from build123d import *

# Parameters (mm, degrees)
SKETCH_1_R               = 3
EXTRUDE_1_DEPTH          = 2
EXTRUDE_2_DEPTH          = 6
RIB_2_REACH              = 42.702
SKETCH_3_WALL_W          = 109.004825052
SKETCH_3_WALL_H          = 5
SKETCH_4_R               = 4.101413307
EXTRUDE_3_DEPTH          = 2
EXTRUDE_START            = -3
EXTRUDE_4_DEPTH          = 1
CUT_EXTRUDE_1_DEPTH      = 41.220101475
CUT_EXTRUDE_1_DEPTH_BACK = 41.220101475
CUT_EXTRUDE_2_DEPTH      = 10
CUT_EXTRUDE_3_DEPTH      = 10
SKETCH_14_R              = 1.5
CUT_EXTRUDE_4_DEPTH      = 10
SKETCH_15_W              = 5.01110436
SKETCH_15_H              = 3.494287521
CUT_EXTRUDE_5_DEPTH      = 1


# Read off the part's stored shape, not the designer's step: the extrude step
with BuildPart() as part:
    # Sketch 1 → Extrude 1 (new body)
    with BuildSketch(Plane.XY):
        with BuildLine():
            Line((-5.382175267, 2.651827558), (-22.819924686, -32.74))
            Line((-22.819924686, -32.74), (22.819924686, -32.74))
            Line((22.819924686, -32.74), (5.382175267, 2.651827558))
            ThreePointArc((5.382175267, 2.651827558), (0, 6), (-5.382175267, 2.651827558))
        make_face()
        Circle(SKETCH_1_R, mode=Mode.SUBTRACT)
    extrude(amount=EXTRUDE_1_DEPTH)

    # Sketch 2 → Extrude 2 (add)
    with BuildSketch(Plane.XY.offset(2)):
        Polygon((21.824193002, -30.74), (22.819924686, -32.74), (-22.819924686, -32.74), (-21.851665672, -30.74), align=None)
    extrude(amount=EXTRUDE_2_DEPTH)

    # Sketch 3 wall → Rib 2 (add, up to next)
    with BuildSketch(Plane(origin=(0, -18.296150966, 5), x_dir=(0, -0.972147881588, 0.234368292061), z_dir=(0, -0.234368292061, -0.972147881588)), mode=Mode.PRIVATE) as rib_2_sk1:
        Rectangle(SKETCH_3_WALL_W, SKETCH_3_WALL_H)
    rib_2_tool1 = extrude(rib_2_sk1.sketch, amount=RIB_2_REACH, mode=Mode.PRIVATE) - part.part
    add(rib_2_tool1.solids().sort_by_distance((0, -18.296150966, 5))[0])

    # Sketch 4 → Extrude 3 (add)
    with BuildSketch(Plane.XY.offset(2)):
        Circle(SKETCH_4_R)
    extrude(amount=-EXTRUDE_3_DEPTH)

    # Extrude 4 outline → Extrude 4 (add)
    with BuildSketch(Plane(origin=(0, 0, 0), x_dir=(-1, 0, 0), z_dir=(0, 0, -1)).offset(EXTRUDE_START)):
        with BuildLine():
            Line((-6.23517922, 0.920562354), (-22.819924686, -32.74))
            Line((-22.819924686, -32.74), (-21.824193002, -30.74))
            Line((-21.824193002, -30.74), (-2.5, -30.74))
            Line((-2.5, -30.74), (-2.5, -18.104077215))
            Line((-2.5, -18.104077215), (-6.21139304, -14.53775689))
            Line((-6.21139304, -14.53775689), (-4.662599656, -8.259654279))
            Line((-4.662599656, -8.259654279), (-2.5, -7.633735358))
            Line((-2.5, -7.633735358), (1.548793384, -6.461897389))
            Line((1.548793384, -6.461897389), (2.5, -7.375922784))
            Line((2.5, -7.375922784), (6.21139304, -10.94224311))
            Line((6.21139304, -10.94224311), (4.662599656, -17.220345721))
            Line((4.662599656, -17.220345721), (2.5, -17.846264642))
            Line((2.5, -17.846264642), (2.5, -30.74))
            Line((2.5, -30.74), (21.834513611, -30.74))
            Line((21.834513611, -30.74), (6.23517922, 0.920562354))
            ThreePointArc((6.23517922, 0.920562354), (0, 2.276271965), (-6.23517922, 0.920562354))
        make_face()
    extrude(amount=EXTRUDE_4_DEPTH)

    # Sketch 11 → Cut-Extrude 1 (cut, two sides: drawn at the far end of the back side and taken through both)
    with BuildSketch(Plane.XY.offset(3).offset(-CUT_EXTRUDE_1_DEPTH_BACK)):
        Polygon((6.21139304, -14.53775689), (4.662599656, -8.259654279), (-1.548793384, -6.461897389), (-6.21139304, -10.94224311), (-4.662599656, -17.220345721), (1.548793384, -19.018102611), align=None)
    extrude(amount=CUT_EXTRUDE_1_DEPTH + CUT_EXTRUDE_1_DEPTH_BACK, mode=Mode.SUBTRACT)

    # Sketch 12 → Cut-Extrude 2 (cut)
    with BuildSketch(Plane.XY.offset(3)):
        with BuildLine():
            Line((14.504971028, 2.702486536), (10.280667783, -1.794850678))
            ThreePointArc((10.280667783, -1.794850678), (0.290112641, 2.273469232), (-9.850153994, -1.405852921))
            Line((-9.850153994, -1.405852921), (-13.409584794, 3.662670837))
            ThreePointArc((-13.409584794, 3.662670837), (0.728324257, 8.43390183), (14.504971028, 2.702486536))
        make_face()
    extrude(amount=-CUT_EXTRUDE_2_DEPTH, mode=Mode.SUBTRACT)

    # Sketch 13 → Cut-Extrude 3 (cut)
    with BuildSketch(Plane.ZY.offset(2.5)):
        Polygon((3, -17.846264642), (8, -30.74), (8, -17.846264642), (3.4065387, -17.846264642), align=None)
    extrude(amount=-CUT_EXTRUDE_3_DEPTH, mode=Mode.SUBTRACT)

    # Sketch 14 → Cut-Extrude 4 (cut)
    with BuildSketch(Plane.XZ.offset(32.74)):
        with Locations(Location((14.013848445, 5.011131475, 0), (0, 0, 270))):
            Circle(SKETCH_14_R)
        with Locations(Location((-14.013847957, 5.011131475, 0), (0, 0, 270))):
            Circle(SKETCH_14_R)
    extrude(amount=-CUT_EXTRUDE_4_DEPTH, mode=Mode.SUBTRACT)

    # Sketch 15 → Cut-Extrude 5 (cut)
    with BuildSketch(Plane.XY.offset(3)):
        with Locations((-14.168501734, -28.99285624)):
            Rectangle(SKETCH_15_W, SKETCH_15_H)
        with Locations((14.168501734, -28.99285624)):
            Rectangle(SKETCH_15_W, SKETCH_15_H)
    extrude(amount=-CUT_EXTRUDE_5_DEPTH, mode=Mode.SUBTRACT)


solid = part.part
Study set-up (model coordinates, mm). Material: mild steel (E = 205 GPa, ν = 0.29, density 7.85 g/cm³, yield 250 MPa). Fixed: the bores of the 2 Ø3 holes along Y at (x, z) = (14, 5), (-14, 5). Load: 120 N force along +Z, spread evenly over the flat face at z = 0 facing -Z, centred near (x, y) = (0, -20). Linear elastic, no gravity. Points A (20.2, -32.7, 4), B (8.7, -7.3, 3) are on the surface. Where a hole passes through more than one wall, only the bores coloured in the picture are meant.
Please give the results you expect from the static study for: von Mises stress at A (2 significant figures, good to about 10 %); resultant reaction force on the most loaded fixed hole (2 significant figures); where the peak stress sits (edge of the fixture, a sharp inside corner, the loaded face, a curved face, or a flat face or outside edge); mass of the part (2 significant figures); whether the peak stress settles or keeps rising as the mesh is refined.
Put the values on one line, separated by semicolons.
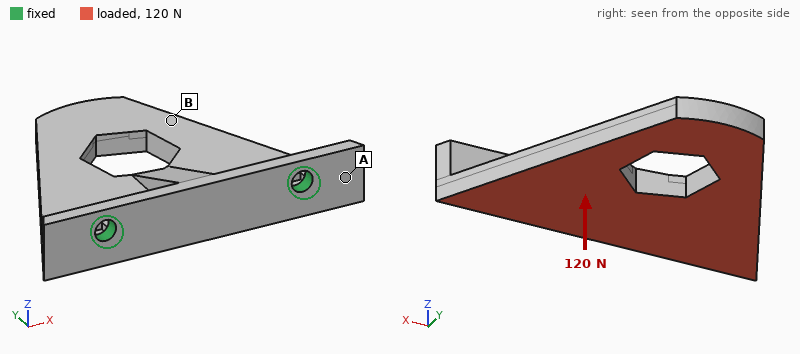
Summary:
28 MPa; 61 N; edge of the fixture; 25 g; keeps rising
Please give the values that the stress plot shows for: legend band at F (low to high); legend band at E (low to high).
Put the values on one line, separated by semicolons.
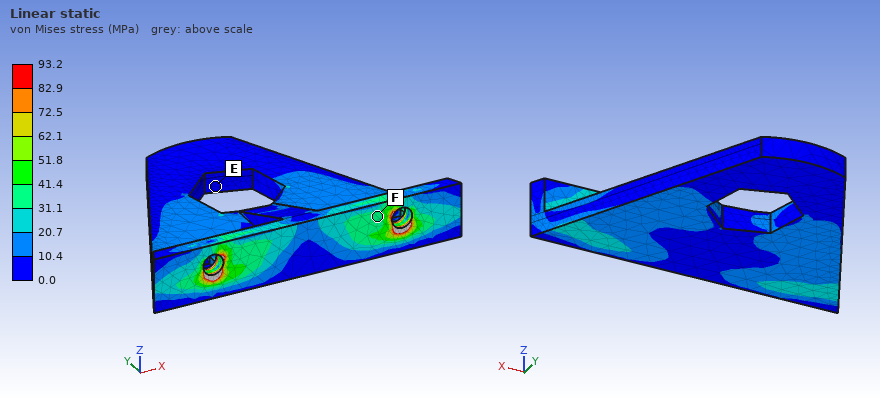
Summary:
31.1 to 41.4 MPa; 0.0 to 10.4 MPa
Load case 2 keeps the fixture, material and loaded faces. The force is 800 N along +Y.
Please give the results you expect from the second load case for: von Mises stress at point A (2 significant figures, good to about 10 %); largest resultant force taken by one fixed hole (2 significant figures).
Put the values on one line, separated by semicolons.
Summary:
44 MPa; 400 N
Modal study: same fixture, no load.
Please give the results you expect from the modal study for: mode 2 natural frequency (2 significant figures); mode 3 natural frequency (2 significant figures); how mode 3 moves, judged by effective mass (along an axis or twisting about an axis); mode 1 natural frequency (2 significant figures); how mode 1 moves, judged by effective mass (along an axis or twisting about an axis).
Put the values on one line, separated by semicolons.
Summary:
8200 Hz; 9600 Hz; along Z; 2000 Hz; along Z
